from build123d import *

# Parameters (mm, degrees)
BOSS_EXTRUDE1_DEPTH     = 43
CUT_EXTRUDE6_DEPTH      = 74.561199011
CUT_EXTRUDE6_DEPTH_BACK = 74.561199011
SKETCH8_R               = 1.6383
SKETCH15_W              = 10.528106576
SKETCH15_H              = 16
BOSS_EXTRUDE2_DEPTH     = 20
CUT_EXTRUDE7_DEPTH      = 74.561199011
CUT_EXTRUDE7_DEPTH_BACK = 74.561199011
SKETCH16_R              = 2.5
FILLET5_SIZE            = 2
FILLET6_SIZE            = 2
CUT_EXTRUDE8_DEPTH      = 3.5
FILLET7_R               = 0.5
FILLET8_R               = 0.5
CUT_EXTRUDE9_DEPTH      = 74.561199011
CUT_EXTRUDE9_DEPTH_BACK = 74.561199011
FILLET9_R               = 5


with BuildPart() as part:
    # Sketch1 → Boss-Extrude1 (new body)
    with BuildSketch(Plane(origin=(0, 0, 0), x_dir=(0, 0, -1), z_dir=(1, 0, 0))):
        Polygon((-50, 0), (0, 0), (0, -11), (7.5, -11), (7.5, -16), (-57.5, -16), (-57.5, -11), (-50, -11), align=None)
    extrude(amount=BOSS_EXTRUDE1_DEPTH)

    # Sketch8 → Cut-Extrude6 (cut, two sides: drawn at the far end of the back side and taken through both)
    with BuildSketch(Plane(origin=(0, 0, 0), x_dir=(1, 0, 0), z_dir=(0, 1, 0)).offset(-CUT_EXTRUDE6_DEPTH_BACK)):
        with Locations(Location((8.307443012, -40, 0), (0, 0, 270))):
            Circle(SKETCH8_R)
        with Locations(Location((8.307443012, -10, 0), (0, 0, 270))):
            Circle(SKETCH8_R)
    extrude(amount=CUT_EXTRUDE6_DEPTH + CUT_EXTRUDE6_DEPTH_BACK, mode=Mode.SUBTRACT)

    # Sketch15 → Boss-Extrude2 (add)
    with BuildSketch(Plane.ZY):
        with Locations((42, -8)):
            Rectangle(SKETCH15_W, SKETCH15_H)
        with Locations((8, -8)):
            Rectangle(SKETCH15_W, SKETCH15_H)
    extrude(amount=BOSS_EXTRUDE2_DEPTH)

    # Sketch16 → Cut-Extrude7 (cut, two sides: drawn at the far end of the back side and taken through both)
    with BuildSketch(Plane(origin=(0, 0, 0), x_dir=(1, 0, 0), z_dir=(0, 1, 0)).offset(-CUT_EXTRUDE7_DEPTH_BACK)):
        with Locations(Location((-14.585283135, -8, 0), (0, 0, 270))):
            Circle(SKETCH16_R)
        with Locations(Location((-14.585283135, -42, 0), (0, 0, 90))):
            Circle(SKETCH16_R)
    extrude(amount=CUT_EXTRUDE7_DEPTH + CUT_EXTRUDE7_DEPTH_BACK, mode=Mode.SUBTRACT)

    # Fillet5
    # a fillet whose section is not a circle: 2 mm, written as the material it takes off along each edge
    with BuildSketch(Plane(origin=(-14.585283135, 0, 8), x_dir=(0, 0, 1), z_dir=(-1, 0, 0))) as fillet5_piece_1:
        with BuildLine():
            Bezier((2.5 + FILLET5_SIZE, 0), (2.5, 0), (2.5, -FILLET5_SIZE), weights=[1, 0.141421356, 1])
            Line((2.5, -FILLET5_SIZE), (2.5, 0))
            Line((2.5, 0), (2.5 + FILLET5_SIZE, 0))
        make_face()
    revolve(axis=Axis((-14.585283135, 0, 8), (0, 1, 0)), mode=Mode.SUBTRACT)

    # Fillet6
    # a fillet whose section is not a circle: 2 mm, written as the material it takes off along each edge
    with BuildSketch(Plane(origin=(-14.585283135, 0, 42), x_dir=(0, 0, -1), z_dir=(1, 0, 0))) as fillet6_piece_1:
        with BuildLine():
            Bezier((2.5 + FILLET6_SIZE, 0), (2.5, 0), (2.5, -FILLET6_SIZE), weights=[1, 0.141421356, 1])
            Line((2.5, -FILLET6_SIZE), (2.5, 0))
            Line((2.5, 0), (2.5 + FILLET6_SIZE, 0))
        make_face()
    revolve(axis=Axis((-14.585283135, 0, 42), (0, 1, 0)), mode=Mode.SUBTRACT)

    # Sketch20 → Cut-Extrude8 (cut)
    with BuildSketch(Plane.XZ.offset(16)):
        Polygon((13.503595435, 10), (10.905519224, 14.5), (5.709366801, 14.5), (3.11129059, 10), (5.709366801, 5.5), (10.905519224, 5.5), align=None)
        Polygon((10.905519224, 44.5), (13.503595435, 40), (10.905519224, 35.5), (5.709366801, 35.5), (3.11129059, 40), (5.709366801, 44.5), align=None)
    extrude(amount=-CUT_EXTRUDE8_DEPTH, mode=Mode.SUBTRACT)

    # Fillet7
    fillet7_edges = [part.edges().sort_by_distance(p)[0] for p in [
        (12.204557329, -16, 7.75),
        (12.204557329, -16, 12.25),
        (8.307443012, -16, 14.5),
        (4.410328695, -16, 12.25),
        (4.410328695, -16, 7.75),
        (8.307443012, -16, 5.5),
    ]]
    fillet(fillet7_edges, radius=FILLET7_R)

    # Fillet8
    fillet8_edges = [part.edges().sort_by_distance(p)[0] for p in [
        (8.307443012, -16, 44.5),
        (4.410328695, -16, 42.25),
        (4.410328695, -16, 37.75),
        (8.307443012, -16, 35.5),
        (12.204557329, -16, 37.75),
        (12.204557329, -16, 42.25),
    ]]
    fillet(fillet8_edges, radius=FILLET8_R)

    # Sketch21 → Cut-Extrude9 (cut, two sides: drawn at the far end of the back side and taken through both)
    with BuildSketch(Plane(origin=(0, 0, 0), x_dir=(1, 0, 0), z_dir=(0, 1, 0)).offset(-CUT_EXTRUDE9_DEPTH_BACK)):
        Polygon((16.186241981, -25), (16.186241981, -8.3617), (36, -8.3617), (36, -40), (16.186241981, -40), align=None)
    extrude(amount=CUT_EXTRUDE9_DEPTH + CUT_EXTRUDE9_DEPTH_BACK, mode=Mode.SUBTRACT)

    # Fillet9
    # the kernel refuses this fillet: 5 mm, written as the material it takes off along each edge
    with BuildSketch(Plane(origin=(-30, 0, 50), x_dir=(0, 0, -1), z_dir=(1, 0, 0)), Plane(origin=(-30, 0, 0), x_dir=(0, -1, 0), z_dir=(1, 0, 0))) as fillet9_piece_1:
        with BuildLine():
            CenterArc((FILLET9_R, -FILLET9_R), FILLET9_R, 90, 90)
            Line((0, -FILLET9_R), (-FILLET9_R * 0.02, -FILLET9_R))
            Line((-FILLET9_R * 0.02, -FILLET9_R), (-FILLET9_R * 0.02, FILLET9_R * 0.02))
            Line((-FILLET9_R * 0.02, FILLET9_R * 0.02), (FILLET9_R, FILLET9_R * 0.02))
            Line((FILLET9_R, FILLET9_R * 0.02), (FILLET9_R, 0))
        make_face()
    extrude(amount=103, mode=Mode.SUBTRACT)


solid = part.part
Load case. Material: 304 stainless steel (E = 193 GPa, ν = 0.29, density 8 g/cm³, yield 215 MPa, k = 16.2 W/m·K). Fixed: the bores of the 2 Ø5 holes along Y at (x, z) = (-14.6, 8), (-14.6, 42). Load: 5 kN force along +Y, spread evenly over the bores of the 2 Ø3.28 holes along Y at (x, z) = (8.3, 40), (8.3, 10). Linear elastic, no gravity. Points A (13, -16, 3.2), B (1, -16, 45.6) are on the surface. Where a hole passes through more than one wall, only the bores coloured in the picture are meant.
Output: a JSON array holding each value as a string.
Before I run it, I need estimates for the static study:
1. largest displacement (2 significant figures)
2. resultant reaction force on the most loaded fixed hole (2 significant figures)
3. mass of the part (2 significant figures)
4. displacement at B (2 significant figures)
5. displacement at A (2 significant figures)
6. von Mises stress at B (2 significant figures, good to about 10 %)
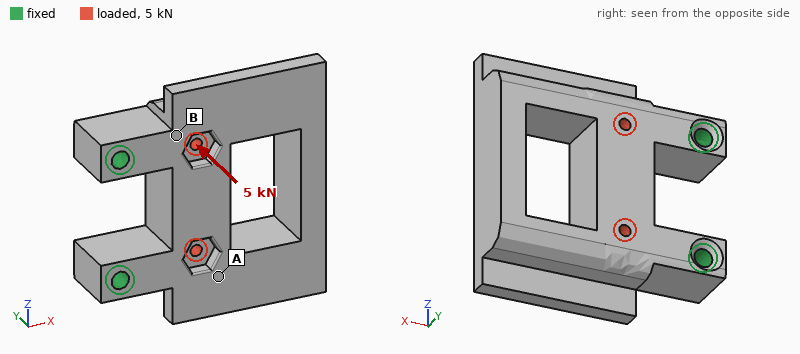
["53 µm", "2.5 kN", "260 g", "13 µm", "24 µm", "34 MPa"]
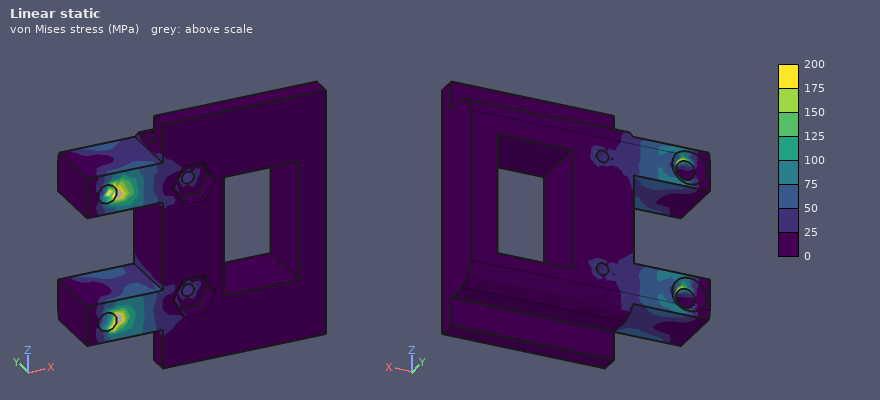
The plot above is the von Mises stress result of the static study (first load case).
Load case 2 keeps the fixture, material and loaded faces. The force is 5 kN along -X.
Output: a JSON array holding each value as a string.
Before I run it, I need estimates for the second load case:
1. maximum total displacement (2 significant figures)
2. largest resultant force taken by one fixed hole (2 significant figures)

["7.6 µm", "2.5 kN"]
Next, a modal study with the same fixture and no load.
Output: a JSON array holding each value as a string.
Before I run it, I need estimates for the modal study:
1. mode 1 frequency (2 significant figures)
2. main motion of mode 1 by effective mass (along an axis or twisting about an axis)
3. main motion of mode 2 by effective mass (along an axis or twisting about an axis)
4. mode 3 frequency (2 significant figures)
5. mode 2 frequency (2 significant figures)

["2700 Hz", "along Y", "along Z", "4900 Hz", "4600 Hz"]
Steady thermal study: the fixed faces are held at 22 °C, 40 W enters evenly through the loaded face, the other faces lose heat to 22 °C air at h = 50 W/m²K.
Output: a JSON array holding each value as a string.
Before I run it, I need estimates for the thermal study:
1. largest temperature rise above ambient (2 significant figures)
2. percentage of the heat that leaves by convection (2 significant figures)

["88 K", "54 %"]
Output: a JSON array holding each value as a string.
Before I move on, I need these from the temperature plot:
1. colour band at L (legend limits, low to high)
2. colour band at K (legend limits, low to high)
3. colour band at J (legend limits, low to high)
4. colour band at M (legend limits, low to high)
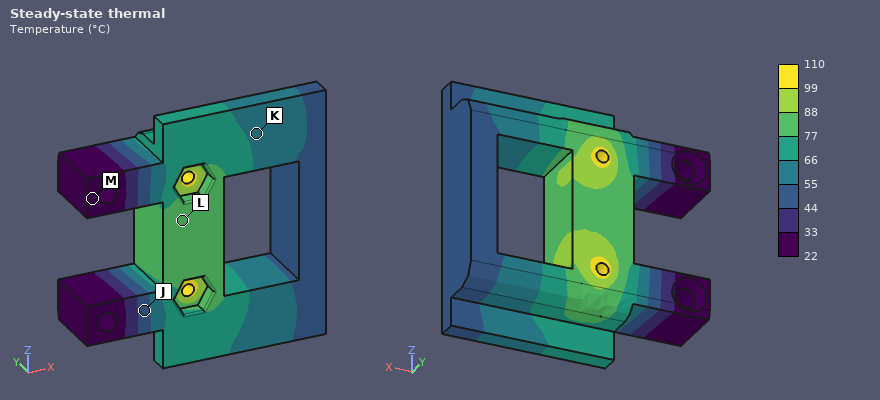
["77 to 88 °C", "55 to 66 °C", "44 to 55 °C", "22 to 33 °C"]
